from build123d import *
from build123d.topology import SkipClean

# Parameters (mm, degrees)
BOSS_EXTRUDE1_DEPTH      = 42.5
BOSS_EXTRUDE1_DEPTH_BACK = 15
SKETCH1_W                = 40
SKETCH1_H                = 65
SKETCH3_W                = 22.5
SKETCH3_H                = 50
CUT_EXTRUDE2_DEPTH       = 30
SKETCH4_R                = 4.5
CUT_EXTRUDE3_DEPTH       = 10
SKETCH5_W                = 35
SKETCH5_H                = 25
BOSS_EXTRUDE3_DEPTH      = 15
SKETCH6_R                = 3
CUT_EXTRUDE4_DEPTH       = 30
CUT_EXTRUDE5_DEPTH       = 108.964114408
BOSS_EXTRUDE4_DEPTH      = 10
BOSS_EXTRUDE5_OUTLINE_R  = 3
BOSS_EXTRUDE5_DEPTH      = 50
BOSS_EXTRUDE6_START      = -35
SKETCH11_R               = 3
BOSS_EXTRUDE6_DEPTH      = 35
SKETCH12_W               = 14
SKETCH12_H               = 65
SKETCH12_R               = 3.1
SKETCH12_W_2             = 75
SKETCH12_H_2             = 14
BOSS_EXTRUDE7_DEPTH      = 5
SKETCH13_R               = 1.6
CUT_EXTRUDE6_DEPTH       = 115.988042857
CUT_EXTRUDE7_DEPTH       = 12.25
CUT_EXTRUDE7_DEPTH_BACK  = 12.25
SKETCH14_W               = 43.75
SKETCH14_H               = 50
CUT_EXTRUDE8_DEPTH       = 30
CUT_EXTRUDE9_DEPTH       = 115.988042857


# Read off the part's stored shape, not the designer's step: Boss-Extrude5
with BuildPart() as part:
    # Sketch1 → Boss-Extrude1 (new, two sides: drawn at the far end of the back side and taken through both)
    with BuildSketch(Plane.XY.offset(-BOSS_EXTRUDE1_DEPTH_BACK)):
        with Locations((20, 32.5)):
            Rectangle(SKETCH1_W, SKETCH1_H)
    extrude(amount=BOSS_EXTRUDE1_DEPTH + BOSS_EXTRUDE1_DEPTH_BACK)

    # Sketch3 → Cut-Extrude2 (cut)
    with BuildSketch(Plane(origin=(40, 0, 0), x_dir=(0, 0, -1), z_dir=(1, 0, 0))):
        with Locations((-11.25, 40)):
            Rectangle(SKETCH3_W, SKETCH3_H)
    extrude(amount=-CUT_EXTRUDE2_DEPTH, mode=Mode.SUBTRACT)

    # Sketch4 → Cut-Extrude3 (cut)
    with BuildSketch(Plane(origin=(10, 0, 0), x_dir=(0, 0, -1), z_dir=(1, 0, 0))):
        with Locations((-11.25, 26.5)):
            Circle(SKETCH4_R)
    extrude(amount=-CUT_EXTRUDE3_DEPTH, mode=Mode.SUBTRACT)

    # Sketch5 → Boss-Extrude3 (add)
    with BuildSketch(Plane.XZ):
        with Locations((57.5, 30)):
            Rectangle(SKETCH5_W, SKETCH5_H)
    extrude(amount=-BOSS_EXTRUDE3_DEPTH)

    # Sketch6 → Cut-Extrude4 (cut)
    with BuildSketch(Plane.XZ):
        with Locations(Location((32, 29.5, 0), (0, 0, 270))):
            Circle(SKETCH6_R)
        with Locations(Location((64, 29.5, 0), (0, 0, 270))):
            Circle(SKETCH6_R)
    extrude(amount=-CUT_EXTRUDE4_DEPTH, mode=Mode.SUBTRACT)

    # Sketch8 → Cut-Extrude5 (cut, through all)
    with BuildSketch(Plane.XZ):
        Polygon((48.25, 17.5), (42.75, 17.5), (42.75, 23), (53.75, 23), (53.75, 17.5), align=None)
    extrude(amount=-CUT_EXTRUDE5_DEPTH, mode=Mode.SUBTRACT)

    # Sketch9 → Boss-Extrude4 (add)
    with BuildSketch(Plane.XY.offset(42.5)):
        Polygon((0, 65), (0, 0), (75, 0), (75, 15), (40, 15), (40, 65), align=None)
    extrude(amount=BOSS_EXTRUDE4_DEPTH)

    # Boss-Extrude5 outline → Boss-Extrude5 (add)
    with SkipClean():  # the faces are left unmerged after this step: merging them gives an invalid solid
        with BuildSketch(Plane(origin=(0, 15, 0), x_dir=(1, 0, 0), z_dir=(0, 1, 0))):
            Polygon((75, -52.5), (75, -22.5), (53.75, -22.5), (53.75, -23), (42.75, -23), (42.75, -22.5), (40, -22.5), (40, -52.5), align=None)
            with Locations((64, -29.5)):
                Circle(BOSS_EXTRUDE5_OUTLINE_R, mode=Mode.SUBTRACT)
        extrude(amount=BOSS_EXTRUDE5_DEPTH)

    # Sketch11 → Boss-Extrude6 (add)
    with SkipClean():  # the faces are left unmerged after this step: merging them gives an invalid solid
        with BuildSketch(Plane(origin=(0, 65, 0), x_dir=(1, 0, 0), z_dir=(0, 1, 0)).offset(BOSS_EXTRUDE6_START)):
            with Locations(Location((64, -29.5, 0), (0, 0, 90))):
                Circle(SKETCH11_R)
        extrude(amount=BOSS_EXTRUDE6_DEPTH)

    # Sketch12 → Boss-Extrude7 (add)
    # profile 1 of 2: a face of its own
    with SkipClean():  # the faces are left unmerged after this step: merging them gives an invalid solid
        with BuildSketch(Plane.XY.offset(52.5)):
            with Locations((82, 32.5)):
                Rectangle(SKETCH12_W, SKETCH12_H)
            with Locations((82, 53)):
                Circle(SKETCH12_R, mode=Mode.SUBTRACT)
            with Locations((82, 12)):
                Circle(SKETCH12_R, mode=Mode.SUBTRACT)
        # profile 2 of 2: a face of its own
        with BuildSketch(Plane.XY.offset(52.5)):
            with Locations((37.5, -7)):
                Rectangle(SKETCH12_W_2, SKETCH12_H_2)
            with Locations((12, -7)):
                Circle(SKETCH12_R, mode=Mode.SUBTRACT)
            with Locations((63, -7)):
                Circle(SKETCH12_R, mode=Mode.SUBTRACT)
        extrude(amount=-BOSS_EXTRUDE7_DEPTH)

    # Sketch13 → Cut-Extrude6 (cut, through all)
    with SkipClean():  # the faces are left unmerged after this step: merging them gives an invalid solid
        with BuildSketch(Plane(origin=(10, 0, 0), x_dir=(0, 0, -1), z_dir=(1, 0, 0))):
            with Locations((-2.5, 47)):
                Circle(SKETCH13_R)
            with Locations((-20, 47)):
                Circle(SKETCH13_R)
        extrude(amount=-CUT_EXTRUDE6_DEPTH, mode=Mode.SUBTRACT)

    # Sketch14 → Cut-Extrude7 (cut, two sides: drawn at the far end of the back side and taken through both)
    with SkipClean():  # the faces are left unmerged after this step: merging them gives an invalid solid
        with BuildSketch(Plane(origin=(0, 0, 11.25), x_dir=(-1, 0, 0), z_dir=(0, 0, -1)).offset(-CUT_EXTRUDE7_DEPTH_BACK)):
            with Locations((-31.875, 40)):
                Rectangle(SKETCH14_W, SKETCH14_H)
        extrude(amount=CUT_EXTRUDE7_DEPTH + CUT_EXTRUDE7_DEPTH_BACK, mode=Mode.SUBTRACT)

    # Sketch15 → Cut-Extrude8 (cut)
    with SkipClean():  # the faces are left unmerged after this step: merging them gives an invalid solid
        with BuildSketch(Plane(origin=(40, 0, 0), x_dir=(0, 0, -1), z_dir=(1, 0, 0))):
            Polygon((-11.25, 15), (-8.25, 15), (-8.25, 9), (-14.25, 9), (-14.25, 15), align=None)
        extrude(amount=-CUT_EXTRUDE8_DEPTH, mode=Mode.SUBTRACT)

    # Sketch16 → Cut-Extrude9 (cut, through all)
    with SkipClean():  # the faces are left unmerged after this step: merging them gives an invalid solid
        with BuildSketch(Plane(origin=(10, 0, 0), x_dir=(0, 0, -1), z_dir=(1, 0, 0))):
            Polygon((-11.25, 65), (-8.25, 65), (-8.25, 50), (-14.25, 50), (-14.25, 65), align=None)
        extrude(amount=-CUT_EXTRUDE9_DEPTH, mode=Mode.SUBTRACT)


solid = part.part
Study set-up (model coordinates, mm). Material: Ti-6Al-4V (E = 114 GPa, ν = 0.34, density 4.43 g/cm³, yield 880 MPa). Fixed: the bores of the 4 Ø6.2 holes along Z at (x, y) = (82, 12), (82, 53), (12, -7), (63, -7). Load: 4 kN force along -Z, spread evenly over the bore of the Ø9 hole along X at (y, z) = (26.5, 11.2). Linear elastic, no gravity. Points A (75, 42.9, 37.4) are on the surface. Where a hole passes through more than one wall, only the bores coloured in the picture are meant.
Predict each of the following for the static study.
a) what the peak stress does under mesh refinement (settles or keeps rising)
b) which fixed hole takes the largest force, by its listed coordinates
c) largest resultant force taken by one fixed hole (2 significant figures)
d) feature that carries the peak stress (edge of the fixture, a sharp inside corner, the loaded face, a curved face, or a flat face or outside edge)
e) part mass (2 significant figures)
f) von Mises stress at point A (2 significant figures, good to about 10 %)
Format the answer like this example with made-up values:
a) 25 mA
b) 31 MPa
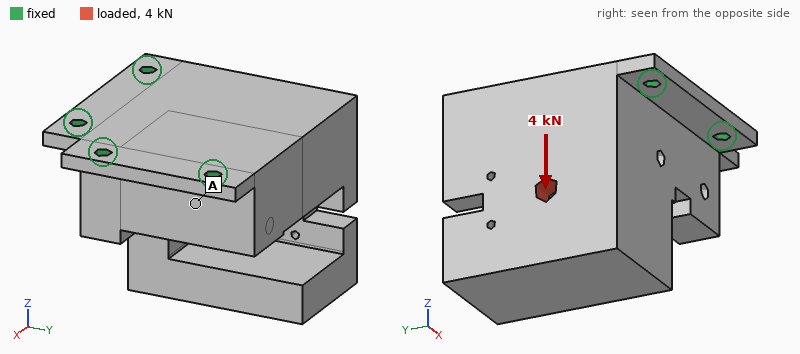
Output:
a) keeps rising
b) (12, -7)
c) 4.9 kN
d) edge of the fixture
e) 940 g
f) 11 MPa
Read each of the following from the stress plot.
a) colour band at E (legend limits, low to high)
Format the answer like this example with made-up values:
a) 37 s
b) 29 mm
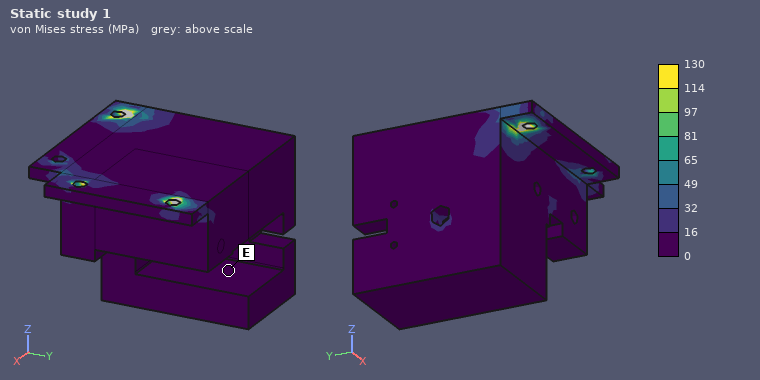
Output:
a) 0 to 16 MPa
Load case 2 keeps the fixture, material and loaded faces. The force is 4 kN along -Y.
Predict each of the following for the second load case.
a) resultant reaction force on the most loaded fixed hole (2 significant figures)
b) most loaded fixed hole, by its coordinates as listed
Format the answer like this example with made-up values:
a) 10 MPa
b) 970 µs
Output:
a) 4.4 kN
b) (82, 53)
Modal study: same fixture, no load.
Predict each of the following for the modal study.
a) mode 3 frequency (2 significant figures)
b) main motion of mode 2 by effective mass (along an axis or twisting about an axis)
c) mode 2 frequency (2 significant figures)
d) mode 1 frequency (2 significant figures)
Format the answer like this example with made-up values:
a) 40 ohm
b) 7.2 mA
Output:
a) 4100 Hz
b) along X
c) 3000 Hz
d) 1400 Hz
